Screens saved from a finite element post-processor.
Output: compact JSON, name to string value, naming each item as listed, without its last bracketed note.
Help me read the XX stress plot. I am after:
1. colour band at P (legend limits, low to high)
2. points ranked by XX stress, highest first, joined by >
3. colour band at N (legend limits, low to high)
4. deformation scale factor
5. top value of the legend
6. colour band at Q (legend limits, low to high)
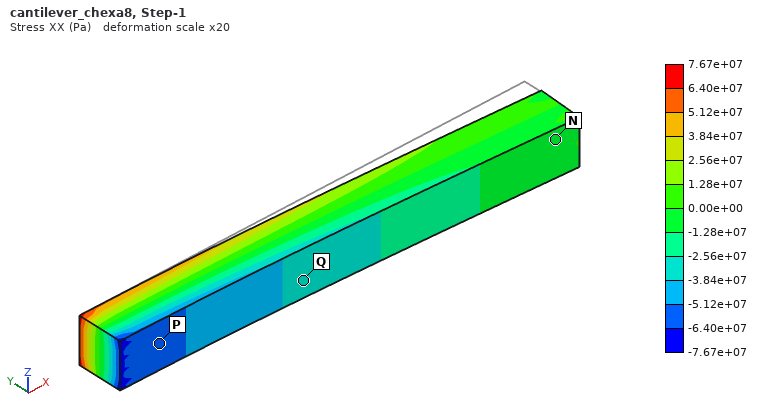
{"colour band at P": "-6.40e+07 to -5.12e+07 Pa", "points ranked by XX stress, highest first, joined by >": "N > Q > P", "colour band at N": "-1.28e+07 to 0.00e+00 Pa", "deformation scale factor": "20", "top value of the legend": "7.67e+07 Pa", "colour band at Q": "-3.84e+07 to -2.56e+07 Pa"}
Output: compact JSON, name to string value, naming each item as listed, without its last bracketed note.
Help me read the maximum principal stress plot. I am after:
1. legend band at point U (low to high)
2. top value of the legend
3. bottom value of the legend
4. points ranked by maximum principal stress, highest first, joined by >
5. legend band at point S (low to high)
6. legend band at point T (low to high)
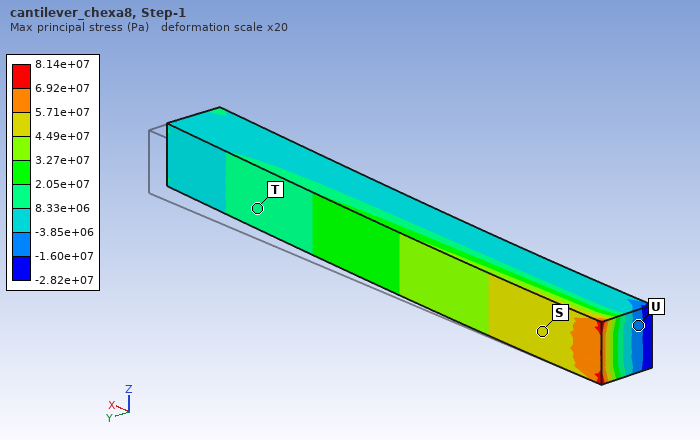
{"legend band at point U": "-1.60e+07 to -3.85e+06 Pa", "top value of the legend": "8.14e+07 Pa", "bottom value of the legend": "-2.82e+07 Pa", "points ranked by maximum principal stress, highest first, joined by >": "S > T > U", "legend band at point S": "4.49e+07 to 5.71e+07 Pa", "legend band at point T": "8.33e+06 to 2.05e+07 Pa"}
